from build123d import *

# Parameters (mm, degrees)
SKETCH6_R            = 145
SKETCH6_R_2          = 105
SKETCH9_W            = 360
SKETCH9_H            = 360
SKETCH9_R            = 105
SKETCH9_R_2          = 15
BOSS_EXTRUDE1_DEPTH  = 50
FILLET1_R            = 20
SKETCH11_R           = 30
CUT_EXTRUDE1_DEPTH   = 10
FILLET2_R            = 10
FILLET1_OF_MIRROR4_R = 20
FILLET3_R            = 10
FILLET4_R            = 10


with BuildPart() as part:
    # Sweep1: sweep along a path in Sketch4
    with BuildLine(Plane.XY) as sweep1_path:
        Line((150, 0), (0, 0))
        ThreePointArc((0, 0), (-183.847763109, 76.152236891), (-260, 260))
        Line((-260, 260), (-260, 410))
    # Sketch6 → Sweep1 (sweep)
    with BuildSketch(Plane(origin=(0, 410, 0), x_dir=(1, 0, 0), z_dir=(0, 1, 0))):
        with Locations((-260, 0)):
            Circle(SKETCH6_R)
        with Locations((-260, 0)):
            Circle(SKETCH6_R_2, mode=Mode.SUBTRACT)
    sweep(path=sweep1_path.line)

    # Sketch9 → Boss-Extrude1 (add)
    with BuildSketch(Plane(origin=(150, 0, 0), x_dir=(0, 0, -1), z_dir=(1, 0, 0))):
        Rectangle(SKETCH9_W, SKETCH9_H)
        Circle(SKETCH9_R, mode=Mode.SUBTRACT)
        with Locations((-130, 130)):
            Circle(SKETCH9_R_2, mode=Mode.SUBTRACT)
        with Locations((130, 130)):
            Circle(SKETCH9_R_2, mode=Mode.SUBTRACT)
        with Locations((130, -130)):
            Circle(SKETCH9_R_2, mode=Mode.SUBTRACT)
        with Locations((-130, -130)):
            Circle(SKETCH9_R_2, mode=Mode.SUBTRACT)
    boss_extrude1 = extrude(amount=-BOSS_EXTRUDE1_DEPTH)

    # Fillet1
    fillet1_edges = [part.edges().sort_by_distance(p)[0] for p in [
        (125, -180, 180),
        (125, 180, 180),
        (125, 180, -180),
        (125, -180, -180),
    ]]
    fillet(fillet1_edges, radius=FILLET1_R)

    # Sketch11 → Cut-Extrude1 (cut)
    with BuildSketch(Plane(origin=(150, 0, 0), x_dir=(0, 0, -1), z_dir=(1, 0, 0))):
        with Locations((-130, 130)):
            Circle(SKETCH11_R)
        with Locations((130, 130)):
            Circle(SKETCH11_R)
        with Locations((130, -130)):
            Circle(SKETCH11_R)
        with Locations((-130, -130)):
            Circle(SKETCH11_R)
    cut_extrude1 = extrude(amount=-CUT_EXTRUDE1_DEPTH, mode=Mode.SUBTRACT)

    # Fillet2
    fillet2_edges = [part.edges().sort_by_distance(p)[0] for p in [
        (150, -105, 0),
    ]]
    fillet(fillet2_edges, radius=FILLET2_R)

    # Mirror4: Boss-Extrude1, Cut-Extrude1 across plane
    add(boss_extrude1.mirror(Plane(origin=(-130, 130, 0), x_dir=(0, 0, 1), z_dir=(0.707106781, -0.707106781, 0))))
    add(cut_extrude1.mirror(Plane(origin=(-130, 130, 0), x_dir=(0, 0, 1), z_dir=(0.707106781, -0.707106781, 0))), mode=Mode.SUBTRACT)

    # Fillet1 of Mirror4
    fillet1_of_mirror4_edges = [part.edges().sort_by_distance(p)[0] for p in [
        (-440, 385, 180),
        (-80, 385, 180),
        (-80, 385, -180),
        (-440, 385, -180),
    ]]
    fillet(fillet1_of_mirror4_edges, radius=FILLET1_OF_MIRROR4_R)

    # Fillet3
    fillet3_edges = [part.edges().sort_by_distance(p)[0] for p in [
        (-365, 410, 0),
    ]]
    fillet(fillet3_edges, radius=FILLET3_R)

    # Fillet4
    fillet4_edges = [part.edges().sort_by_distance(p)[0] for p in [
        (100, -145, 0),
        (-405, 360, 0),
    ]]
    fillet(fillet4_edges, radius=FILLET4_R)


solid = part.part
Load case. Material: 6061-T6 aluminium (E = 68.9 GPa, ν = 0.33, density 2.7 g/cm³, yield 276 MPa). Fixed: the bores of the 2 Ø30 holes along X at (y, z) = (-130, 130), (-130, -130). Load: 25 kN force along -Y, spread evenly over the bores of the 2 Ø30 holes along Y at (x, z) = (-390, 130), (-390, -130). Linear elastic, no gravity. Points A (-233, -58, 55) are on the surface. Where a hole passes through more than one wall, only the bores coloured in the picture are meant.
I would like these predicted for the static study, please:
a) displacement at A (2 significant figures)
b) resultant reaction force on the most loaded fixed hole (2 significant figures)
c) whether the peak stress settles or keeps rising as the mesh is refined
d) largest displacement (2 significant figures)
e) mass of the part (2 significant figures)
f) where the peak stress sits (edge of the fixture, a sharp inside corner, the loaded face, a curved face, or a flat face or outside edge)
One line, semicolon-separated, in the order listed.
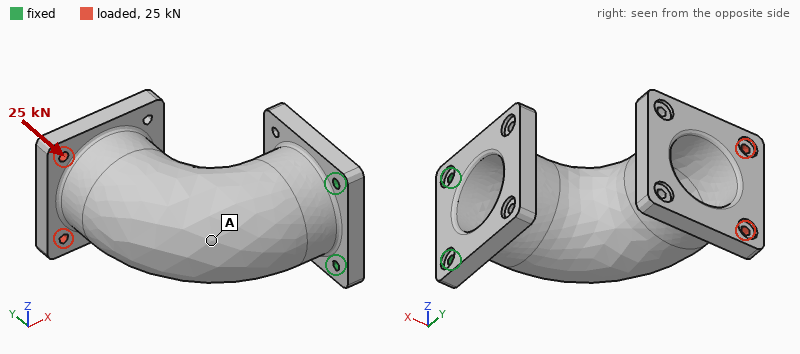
1.8 mm; 13 kN; keeps rising; 3.8 mm; 76 kg; edge of the fixture
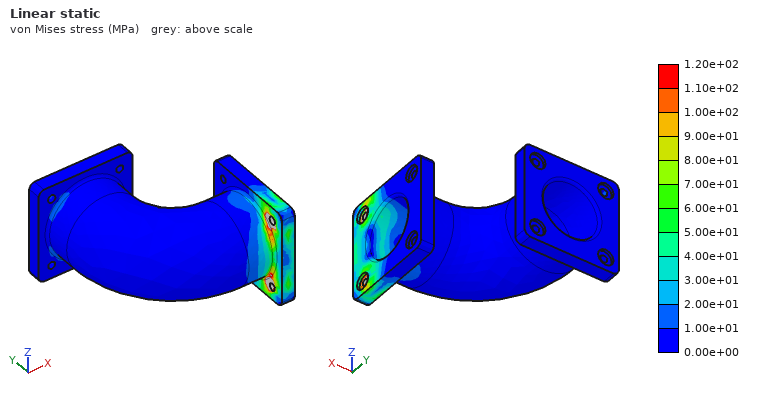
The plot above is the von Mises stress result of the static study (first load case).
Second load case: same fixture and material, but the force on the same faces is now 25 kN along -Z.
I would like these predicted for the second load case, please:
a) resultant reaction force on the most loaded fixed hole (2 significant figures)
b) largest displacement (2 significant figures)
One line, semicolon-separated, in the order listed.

70 kN; 0.60 mm
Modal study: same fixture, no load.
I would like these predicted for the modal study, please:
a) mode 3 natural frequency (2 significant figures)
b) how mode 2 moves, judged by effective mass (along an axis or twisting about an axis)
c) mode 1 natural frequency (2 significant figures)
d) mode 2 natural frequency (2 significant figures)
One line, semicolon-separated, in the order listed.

540 Hz; along Z; 70 Hz; 220 Hz
